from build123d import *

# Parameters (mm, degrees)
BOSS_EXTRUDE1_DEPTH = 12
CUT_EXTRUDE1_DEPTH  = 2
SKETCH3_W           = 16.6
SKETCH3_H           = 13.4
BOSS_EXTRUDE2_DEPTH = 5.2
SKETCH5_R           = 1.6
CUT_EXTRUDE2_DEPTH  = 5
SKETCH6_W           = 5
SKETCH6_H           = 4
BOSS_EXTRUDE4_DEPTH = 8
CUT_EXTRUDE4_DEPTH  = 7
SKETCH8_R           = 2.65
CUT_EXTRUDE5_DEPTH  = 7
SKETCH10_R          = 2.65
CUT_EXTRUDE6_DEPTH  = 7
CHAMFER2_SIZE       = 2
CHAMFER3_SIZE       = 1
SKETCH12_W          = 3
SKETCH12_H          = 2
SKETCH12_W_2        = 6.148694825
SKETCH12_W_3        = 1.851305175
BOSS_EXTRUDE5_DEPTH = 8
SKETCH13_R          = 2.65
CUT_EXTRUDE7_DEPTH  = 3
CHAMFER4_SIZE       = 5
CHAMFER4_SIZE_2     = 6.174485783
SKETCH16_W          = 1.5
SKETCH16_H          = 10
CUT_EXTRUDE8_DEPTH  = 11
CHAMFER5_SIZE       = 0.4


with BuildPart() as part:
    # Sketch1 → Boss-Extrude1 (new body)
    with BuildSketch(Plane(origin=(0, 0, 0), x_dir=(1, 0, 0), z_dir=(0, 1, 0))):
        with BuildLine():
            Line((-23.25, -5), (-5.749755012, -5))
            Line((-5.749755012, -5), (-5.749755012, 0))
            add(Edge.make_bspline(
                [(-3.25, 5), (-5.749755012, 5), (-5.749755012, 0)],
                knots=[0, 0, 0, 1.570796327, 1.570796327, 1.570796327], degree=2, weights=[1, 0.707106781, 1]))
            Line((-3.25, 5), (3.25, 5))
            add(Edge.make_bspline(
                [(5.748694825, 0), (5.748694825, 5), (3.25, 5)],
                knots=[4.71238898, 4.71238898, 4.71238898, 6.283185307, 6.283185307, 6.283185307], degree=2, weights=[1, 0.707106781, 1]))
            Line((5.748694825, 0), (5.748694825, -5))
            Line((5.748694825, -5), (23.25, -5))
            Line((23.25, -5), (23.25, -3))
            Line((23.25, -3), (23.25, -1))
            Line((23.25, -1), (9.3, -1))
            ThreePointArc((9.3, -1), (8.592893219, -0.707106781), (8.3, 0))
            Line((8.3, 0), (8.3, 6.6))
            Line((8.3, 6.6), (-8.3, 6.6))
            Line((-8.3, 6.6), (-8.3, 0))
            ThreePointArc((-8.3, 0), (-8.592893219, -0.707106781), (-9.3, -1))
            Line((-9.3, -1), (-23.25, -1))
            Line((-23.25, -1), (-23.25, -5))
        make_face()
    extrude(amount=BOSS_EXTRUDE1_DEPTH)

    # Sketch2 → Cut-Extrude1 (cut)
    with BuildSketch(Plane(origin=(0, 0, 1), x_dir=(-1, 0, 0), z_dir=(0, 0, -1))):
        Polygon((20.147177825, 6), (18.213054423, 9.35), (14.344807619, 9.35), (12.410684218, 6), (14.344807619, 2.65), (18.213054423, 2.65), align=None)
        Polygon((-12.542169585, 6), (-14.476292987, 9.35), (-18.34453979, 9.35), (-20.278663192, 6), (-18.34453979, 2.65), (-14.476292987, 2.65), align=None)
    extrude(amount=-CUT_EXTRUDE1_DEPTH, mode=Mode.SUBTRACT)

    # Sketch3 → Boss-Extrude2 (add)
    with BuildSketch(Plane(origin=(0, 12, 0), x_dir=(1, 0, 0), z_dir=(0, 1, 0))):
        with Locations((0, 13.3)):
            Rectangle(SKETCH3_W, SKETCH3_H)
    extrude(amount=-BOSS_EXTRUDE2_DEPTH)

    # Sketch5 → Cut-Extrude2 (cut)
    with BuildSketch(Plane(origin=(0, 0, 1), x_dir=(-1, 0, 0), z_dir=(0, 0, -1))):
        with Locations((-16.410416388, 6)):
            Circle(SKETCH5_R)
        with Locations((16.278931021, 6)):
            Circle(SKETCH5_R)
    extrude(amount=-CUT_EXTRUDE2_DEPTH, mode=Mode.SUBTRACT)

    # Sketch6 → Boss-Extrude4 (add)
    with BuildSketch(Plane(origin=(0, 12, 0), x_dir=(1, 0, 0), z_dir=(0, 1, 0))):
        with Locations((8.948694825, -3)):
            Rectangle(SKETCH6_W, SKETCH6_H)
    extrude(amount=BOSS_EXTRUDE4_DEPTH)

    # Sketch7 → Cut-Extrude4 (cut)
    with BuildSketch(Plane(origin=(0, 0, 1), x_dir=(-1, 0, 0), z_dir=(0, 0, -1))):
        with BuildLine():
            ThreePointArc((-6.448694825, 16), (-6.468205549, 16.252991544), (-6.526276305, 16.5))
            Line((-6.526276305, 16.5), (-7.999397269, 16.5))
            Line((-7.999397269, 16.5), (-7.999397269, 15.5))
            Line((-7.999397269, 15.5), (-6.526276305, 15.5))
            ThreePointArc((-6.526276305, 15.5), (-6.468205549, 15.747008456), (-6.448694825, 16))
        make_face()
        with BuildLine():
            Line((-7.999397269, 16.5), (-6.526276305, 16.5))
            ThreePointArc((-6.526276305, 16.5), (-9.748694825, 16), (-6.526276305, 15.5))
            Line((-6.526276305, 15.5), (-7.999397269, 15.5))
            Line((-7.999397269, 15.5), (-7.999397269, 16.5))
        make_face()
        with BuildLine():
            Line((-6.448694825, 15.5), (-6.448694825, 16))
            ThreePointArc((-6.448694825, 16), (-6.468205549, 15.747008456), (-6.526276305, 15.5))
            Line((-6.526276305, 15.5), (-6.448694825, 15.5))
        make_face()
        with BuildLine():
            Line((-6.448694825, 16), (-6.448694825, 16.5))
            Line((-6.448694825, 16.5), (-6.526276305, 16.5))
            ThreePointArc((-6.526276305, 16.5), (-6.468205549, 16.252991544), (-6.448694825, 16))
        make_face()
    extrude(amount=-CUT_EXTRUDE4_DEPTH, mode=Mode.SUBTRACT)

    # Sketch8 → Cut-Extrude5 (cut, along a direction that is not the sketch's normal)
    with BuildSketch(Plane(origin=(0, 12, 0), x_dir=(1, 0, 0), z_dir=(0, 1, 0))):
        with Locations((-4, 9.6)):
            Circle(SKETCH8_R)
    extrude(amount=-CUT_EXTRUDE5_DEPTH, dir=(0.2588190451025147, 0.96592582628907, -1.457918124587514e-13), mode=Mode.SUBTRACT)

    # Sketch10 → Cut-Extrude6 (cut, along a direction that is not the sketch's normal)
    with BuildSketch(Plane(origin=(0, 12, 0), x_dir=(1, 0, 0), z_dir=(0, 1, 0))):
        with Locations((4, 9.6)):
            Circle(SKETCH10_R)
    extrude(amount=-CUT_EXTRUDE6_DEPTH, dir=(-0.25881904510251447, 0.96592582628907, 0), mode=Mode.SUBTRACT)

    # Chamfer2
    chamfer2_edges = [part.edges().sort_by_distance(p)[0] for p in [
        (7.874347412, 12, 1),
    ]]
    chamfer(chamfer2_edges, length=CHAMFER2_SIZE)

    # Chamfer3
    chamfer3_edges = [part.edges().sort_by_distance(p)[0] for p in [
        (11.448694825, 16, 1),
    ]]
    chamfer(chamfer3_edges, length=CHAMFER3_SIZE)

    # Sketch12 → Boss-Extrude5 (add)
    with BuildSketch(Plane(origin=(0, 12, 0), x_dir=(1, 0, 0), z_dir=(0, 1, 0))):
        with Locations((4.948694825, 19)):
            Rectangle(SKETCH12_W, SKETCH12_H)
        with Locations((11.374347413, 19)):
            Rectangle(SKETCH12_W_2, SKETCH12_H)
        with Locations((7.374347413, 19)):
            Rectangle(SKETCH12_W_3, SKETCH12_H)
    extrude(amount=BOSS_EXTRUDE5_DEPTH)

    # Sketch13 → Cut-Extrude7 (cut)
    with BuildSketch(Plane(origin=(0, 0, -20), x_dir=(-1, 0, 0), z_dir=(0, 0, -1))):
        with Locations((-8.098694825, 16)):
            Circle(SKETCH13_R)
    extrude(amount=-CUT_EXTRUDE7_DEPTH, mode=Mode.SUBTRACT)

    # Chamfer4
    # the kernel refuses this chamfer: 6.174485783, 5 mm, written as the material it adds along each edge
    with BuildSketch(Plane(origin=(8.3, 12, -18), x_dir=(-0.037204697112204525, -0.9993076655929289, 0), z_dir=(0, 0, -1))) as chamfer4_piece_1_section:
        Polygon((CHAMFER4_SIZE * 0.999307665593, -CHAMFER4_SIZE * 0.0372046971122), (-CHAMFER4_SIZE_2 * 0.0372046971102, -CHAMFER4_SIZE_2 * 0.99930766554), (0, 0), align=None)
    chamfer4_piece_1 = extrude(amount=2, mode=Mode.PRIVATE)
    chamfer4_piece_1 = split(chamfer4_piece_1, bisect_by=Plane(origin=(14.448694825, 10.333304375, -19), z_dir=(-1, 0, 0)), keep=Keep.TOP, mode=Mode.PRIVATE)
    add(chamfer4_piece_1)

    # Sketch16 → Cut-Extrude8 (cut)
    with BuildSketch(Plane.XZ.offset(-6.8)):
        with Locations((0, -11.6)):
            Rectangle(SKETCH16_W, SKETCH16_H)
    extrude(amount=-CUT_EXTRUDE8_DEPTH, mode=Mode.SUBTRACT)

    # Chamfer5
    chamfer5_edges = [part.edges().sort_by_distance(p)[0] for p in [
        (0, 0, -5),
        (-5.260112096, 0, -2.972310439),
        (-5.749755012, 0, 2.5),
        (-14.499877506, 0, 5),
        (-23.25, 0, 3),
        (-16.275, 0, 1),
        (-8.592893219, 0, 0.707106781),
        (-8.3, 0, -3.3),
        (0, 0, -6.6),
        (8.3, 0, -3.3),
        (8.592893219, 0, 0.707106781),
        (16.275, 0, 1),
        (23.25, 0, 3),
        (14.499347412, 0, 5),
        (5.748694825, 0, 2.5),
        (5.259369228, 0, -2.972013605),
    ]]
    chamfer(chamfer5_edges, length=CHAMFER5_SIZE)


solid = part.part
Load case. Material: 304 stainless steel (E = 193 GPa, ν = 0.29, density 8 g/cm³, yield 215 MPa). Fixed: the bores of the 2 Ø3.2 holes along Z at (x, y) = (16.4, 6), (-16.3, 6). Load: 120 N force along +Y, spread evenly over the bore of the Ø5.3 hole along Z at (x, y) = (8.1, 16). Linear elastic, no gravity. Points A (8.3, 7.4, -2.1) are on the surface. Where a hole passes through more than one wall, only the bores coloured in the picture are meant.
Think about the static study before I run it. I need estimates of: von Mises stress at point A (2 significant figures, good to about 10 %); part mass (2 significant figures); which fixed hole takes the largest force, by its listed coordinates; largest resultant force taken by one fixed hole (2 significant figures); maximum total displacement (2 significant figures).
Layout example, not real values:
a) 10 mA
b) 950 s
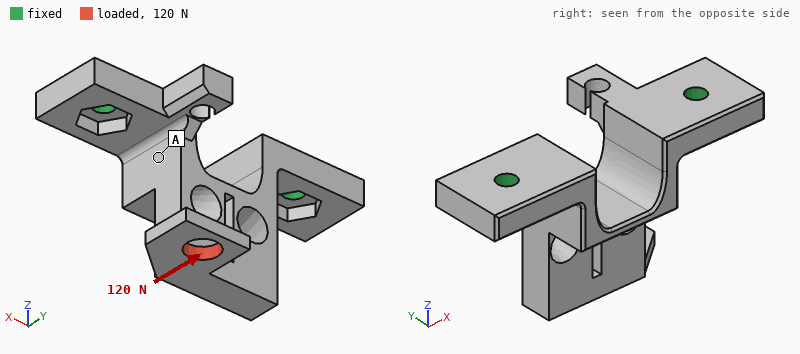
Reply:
a) 16 MPa
b) 27 g
c) (16.4, 6)
d) 84 N
e) 70 µm
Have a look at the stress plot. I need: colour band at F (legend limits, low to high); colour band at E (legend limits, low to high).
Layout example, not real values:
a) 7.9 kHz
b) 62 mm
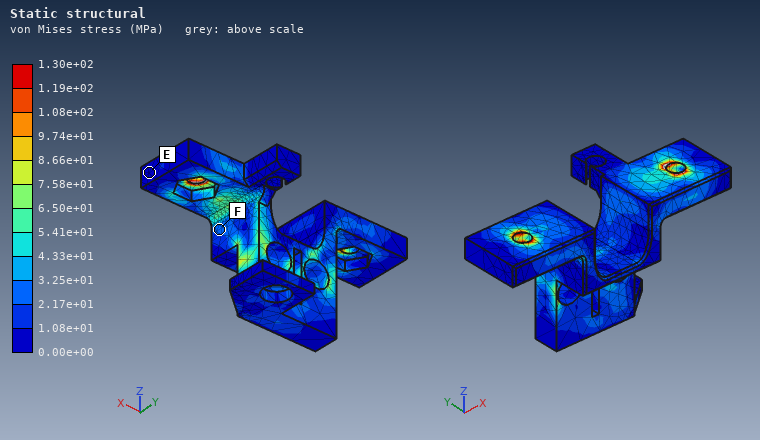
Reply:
a) 2.17e+01 to 3.25e+01 MPa
b) 0.00e+00 to 1.08e+01 MPa
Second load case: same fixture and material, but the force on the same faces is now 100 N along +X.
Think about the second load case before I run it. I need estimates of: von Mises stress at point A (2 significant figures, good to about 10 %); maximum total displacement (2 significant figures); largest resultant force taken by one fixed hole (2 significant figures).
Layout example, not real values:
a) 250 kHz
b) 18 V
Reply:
a) 22 MPa
b) 22 µm
c) 110 N
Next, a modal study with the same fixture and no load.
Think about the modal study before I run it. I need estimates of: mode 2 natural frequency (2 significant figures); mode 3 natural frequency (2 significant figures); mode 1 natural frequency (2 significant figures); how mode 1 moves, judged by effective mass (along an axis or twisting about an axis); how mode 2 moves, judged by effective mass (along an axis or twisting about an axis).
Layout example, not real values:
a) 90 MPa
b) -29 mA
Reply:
a) 7200 Hz
b) 8800 Hz
c) 3300 Hz
d) along Y
e) along X
